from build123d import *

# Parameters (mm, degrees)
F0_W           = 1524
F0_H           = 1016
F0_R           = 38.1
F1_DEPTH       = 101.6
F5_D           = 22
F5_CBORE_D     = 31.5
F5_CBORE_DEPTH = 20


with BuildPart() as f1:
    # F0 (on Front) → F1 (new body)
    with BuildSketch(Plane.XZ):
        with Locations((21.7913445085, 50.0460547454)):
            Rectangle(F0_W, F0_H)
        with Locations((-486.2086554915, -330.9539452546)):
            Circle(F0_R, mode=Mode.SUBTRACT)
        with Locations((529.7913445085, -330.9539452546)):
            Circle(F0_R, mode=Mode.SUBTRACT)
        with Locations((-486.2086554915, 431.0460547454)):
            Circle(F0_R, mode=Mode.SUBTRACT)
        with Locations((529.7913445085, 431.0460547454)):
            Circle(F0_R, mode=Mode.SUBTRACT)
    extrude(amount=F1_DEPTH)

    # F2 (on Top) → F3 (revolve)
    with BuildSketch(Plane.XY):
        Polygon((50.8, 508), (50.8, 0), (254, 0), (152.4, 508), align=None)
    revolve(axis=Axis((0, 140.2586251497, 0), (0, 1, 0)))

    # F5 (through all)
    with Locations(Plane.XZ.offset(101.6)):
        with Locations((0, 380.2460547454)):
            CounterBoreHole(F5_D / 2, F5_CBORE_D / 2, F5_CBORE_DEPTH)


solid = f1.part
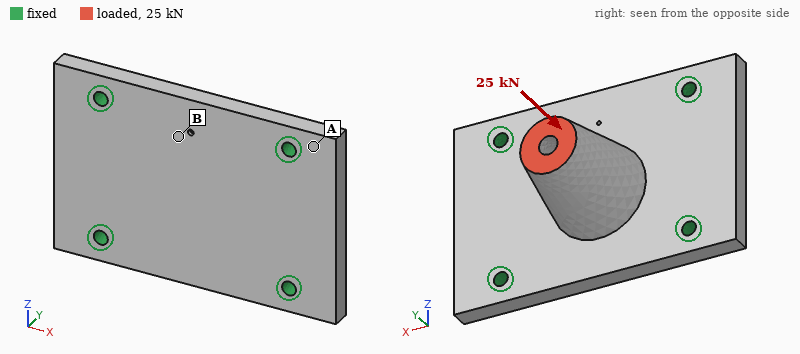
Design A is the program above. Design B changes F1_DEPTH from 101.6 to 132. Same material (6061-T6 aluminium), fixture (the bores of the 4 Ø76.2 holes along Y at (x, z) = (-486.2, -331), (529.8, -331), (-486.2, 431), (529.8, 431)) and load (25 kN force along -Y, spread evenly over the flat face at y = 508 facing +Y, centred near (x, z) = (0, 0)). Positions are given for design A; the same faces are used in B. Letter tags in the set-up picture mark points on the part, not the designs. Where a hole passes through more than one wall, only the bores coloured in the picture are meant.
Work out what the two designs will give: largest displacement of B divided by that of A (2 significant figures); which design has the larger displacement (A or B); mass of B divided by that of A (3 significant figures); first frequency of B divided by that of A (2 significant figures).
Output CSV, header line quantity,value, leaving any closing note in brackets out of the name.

quantity,value
largest displacement of B divided by that of A,0.58
which design has the larger displacement,A
mass of B divided by that of A,1.21
first frequency of B divided by that of A,1.3
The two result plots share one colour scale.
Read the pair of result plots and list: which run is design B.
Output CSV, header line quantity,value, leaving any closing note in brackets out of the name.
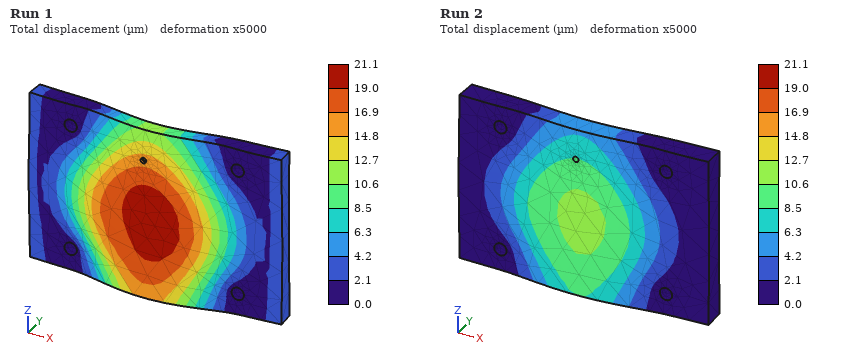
quantity,value
which run is design B,Run 2
